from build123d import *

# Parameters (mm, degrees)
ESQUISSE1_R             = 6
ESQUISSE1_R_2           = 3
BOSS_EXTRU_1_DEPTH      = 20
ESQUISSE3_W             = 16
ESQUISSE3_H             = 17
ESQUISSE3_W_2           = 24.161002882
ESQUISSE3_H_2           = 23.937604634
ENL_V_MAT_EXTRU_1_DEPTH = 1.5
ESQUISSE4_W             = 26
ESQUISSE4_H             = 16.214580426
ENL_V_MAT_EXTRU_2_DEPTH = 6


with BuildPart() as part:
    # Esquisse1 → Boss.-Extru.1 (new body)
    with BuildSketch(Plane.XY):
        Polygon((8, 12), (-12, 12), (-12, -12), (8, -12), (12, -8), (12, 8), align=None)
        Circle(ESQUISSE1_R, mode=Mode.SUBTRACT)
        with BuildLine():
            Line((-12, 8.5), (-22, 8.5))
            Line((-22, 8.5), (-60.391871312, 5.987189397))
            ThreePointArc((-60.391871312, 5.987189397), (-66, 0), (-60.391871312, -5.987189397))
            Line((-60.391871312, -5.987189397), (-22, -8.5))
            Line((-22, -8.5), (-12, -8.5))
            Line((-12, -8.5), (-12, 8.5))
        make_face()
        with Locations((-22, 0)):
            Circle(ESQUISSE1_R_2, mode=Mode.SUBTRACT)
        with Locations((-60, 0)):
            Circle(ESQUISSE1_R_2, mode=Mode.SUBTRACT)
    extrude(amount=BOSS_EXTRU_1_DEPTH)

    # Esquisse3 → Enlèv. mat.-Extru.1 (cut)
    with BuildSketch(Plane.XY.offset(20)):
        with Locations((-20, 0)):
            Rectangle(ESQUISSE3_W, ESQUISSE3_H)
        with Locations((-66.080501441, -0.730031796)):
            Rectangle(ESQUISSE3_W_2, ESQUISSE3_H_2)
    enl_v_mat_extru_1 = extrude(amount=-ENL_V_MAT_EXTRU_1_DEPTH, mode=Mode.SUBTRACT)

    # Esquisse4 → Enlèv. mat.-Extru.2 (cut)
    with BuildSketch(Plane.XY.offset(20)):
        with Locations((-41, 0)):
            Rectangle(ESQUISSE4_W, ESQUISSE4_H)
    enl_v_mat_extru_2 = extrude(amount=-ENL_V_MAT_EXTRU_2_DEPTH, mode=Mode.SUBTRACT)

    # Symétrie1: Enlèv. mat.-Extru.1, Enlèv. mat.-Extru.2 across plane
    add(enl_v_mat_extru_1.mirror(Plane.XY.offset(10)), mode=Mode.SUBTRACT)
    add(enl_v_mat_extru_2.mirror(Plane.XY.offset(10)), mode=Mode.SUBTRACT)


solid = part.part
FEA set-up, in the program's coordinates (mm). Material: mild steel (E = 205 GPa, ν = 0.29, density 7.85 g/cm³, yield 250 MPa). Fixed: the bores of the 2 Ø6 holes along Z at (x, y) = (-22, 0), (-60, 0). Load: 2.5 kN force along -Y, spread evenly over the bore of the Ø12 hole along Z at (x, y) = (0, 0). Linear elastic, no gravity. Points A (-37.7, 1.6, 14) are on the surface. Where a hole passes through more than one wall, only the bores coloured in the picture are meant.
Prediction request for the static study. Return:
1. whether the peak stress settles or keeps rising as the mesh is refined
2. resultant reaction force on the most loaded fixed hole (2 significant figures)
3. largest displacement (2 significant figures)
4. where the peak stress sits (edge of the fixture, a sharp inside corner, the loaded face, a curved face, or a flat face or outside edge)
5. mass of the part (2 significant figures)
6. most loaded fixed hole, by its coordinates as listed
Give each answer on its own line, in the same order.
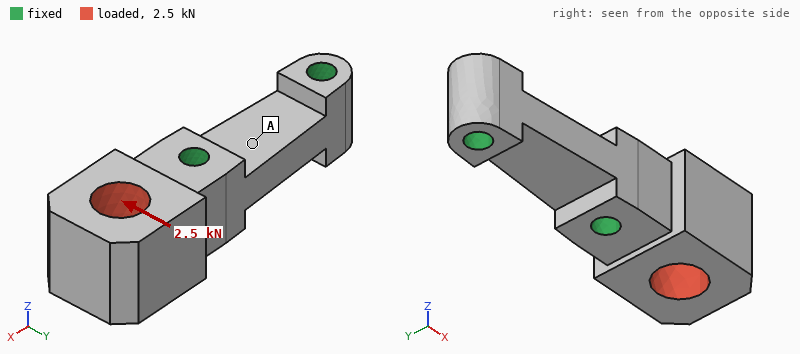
keeps rising
2.8 kN
23 µm
edge of the fixture
140 g
(-22, 0)
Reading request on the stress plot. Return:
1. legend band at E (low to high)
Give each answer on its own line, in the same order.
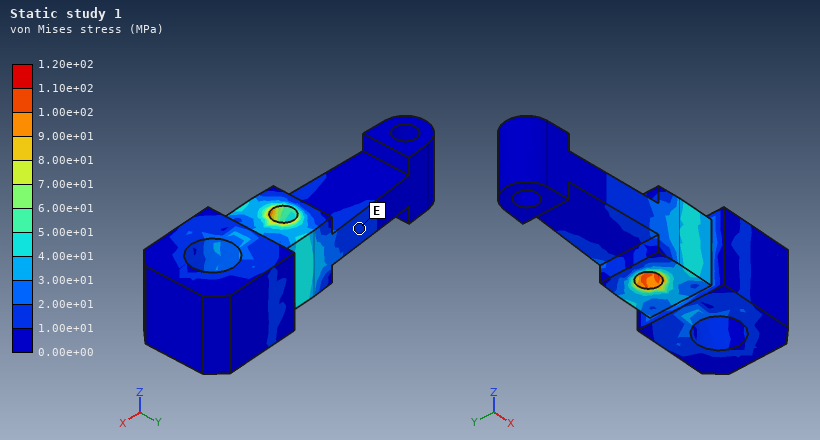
1.00e+01 to 2.00e+01 MPa
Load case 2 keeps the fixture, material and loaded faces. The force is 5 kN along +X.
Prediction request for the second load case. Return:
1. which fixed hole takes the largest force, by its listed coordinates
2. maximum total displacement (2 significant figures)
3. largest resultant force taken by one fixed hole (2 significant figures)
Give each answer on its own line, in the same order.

(-22, 0)
3.4 µm
4.9 kN
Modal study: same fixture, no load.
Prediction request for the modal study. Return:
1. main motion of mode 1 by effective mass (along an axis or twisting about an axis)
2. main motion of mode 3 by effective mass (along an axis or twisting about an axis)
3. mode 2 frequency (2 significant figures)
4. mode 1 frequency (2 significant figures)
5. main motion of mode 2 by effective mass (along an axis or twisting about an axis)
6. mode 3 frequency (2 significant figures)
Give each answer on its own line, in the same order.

along Y
twisting about X
9300 Hz
7300 Hz
along Z
16 kHz
